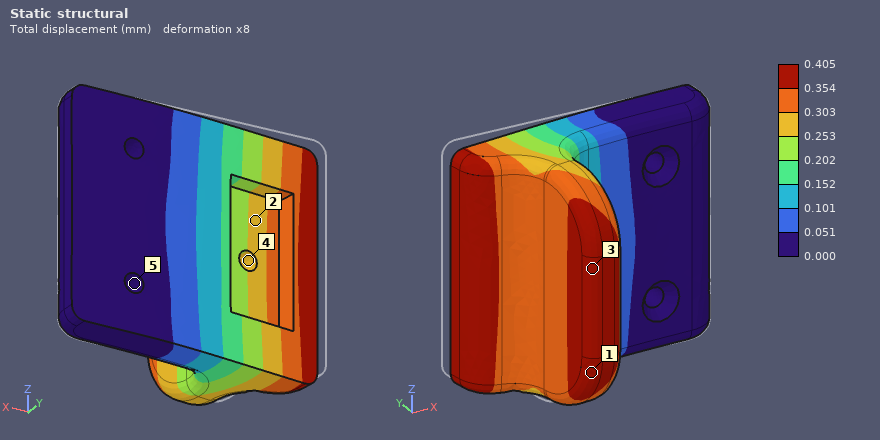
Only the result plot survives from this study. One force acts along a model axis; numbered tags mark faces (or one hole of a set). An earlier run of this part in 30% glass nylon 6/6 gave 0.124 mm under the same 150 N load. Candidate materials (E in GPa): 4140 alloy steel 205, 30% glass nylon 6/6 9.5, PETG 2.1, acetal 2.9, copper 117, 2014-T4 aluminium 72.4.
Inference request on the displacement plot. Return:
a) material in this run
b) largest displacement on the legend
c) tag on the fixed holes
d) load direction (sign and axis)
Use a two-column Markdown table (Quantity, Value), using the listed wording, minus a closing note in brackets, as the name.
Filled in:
| Quantity | Value |
|---|---|
| material in this run | acetal |
| largest displacement on the legend | 0.405 mm |
| tag on the fixed holes | 5 |
| load direction | -Y |
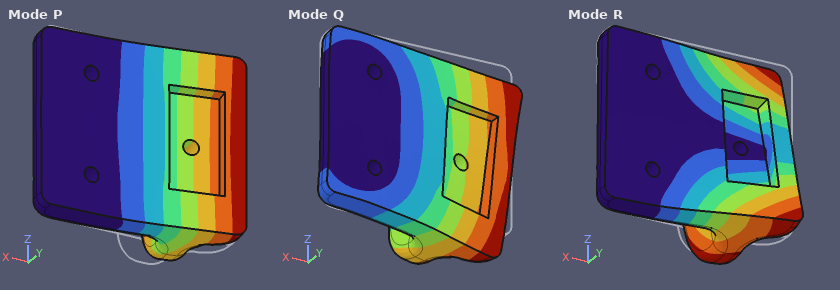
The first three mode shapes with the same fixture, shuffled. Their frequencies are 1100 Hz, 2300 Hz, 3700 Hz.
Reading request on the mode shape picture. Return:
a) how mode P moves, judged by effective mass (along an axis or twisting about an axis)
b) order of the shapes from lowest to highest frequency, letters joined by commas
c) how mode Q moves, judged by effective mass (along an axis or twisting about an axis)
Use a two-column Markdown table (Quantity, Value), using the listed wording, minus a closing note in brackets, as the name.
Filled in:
| Quantity | Value |
|---|---|
| how mode P moves, judged by effective mass | along Y |
| order of the shapes from lowest to highest frequency, letters joined by commas | P, R, Q |
| how mode Q moves, judged by effective mass | along Z |
